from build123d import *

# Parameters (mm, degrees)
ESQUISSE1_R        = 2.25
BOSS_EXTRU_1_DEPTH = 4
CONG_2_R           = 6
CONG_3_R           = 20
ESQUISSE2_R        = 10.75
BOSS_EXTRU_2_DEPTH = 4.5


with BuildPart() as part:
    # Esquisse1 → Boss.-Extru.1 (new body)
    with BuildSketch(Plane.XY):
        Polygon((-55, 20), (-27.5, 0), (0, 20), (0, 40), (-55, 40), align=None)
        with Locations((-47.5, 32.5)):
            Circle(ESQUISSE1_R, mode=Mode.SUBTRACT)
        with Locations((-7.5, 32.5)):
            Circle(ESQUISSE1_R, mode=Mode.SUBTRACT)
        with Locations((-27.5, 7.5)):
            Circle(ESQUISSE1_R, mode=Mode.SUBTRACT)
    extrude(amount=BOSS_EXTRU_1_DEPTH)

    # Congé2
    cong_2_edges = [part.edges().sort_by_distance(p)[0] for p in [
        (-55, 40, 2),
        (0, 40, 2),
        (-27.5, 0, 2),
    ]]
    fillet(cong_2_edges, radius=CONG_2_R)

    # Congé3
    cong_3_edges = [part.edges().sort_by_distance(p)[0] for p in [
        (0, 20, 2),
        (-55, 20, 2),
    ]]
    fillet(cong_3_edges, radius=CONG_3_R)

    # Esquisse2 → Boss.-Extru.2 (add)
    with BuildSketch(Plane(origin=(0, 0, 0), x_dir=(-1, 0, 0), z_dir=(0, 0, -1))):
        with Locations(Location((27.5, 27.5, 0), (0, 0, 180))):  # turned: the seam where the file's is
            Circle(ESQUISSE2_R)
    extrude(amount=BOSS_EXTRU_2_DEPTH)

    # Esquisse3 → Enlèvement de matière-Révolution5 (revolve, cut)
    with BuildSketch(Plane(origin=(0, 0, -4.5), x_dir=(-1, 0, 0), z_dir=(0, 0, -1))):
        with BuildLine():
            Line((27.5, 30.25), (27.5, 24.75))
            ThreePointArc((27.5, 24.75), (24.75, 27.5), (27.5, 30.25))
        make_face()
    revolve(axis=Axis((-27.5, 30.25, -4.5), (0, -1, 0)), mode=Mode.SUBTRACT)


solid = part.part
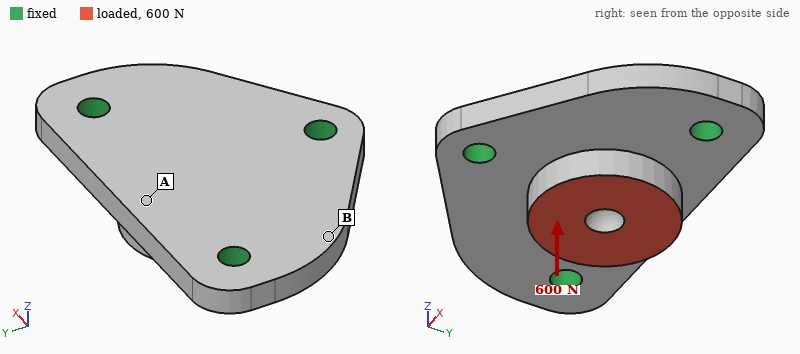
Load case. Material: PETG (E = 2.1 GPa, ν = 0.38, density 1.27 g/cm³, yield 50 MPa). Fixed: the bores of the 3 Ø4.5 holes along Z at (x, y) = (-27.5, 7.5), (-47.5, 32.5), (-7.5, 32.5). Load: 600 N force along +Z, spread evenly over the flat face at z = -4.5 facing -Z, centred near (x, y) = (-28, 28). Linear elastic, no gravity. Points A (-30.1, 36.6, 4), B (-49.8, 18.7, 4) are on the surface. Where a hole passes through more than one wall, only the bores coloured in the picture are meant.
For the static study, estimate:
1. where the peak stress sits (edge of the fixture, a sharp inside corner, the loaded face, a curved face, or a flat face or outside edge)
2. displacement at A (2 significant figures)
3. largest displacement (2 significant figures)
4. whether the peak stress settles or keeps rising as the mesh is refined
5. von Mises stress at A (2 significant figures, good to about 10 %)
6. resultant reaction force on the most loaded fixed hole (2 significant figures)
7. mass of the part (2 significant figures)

edge of the fixture
0.30 mm
0.34 mm
keeps rising
9.3 MPa
250 N
9.9 g
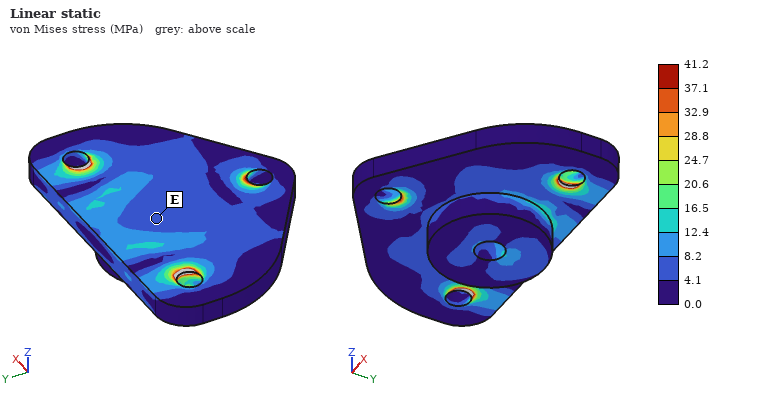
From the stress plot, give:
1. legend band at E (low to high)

4.1 to 8.2 MPa
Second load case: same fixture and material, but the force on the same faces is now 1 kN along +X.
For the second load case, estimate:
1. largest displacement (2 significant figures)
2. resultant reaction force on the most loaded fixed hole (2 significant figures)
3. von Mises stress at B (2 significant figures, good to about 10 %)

0.18 mm
450 N
4.1 MPa
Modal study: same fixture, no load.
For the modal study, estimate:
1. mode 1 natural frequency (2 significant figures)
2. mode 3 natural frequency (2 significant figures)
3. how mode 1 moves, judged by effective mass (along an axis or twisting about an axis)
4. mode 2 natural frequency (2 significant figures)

3600 Hz
4700 Hz
along Z
4600 Hz
